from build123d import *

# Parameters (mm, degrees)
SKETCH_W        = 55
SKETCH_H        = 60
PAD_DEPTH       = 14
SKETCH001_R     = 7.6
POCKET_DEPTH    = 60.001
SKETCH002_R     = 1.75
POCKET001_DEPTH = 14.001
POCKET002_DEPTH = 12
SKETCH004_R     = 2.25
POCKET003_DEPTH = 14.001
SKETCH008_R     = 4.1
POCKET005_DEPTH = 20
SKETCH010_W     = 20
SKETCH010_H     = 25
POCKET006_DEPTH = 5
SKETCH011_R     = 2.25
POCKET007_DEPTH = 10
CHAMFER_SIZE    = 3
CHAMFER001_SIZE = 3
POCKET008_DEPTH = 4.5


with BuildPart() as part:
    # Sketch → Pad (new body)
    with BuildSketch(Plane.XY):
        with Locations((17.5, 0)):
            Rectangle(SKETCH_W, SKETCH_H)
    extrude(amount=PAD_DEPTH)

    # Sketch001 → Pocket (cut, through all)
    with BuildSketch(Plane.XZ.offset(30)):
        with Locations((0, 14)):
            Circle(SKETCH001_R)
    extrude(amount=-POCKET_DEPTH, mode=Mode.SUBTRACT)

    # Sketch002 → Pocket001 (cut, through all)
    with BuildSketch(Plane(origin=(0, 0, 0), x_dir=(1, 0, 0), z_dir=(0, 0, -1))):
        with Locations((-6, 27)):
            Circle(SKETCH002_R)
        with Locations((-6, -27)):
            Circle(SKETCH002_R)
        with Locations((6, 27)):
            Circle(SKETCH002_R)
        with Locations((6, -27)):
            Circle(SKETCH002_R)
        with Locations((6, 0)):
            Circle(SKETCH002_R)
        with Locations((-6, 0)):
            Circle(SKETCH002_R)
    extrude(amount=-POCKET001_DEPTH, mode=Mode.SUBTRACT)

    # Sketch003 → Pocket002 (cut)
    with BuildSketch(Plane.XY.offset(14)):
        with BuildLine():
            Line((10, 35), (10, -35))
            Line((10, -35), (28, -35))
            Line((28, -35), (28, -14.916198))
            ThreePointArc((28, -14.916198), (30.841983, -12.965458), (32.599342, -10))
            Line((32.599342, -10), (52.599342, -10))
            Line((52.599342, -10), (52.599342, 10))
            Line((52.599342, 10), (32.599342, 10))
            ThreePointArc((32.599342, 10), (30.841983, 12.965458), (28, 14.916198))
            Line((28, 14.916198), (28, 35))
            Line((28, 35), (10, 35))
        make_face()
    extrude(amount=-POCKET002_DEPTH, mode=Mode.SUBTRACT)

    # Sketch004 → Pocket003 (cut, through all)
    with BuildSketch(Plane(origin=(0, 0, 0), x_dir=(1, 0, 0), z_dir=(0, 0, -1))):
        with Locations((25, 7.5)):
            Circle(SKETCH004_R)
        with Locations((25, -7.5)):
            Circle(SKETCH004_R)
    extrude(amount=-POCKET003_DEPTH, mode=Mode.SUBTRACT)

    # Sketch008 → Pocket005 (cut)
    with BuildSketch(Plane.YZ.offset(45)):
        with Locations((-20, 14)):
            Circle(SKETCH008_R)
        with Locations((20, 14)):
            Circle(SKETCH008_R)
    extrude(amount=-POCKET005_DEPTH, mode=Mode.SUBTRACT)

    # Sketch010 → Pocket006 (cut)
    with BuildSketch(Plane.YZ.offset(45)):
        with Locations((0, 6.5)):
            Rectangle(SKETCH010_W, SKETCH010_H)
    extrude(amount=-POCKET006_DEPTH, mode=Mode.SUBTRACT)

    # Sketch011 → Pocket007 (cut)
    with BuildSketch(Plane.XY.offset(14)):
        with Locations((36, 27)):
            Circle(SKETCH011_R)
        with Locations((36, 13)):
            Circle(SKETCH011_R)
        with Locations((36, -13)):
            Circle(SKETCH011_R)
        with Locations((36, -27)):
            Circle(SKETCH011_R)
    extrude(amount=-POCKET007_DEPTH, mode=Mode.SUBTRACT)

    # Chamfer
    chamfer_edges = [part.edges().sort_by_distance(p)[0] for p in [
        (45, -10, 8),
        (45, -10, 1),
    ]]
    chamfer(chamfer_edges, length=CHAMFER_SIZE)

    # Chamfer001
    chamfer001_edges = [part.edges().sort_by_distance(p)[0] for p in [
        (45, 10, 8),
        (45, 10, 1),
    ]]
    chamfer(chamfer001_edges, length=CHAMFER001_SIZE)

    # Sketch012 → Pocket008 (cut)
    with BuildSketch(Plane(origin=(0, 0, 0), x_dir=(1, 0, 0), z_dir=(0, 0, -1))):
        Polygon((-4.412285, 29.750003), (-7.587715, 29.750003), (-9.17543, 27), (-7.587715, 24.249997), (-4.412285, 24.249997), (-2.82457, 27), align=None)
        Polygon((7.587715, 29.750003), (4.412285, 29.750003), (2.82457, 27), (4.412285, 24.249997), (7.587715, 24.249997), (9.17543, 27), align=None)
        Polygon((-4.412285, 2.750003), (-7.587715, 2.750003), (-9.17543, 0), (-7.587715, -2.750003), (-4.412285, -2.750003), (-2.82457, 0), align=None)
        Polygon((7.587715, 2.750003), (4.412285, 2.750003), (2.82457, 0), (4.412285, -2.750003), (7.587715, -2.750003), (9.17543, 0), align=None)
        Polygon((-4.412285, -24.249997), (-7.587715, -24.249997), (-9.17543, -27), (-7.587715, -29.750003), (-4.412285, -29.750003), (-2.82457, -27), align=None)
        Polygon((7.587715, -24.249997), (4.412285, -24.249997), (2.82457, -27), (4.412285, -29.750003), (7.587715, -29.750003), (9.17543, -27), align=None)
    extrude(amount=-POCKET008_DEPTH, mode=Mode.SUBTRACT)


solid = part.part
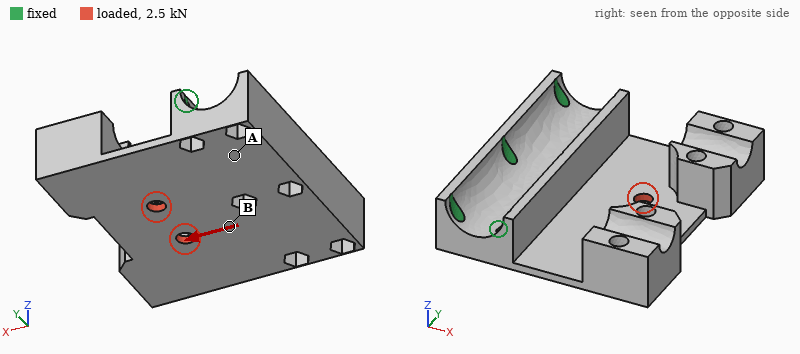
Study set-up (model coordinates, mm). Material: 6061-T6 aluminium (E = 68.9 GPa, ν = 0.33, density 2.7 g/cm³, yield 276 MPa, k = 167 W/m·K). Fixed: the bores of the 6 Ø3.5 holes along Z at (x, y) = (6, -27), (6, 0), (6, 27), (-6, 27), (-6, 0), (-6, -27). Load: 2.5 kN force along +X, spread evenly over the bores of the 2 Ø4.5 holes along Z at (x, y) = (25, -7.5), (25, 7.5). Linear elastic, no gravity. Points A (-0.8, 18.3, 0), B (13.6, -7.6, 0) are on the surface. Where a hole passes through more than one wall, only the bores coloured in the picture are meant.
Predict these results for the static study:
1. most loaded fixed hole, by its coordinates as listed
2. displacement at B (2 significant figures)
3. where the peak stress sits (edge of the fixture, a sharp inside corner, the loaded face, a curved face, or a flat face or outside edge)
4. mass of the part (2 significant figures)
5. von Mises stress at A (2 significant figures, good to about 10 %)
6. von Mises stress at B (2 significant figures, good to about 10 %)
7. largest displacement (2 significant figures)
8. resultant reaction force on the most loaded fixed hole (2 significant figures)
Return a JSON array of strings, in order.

["(6, 0)", "9.6 µm", "the loaded face", "55 g", "7.9 MPa", "34 MPa", "35 µm", "840 N"]
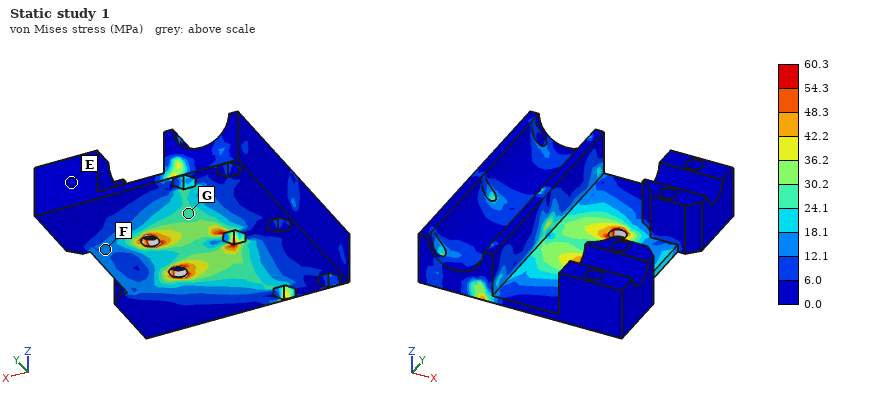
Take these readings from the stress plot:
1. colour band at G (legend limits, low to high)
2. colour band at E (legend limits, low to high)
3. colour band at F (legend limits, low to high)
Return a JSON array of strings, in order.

["24.1 to 30.2 MPa", "0.0 to 6.0 MPa", "12.1 to 18.1 MPa"]
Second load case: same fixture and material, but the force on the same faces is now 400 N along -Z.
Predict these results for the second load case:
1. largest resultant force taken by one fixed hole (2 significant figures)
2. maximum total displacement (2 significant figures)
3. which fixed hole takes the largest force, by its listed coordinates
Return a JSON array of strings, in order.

["560 N", "0.60 mm", "(6, 0)"]
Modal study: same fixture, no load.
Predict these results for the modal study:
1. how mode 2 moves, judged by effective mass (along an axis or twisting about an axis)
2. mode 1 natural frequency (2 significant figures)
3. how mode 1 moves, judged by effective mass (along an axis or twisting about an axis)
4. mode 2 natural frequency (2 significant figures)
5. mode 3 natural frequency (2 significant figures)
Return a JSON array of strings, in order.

["twisting about X", "640 Hz", "along Z", "1000 Hz", "2500 Hz"]
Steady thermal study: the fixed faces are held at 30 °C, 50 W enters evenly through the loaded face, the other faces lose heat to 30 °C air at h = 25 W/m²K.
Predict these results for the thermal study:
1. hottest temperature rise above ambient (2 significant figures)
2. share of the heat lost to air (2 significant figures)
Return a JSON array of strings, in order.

["61 K", "12 %"]
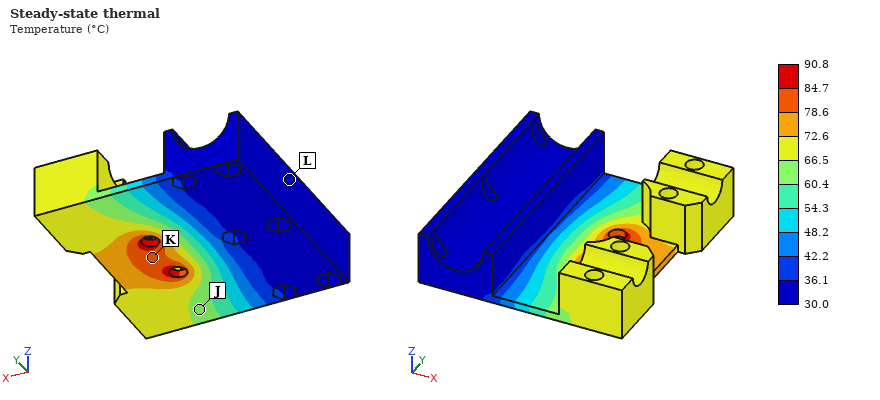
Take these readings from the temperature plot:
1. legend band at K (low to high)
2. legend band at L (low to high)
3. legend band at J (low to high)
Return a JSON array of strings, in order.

["78.6 to 84.7 °C", "30.0 to 36.1 °C", "60.4 to 66.5 °C"]
